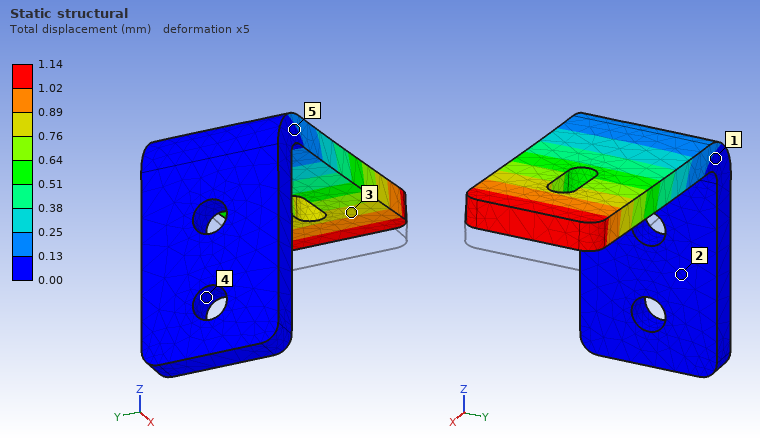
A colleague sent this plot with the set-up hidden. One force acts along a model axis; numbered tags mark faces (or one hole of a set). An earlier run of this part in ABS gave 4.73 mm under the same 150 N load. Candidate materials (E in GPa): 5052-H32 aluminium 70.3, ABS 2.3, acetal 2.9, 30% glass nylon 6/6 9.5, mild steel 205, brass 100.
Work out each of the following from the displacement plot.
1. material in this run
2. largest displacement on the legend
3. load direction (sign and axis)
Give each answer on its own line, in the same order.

30% glass nylon 6/6
1.14 mm
+Z
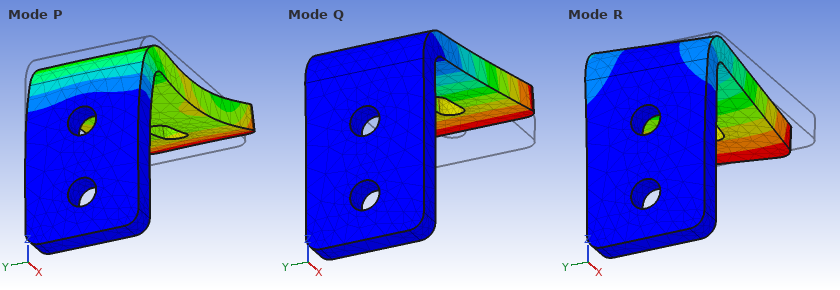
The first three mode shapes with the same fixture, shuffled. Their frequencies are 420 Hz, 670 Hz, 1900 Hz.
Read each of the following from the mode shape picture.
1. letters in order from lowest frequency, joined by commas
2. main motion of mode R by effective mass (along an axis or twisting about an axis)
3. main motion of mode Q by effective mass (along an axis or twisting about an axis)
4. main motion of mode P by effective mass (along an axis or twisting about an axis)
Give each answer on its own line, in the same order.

Q, R, P
along Y
along Z
along X
